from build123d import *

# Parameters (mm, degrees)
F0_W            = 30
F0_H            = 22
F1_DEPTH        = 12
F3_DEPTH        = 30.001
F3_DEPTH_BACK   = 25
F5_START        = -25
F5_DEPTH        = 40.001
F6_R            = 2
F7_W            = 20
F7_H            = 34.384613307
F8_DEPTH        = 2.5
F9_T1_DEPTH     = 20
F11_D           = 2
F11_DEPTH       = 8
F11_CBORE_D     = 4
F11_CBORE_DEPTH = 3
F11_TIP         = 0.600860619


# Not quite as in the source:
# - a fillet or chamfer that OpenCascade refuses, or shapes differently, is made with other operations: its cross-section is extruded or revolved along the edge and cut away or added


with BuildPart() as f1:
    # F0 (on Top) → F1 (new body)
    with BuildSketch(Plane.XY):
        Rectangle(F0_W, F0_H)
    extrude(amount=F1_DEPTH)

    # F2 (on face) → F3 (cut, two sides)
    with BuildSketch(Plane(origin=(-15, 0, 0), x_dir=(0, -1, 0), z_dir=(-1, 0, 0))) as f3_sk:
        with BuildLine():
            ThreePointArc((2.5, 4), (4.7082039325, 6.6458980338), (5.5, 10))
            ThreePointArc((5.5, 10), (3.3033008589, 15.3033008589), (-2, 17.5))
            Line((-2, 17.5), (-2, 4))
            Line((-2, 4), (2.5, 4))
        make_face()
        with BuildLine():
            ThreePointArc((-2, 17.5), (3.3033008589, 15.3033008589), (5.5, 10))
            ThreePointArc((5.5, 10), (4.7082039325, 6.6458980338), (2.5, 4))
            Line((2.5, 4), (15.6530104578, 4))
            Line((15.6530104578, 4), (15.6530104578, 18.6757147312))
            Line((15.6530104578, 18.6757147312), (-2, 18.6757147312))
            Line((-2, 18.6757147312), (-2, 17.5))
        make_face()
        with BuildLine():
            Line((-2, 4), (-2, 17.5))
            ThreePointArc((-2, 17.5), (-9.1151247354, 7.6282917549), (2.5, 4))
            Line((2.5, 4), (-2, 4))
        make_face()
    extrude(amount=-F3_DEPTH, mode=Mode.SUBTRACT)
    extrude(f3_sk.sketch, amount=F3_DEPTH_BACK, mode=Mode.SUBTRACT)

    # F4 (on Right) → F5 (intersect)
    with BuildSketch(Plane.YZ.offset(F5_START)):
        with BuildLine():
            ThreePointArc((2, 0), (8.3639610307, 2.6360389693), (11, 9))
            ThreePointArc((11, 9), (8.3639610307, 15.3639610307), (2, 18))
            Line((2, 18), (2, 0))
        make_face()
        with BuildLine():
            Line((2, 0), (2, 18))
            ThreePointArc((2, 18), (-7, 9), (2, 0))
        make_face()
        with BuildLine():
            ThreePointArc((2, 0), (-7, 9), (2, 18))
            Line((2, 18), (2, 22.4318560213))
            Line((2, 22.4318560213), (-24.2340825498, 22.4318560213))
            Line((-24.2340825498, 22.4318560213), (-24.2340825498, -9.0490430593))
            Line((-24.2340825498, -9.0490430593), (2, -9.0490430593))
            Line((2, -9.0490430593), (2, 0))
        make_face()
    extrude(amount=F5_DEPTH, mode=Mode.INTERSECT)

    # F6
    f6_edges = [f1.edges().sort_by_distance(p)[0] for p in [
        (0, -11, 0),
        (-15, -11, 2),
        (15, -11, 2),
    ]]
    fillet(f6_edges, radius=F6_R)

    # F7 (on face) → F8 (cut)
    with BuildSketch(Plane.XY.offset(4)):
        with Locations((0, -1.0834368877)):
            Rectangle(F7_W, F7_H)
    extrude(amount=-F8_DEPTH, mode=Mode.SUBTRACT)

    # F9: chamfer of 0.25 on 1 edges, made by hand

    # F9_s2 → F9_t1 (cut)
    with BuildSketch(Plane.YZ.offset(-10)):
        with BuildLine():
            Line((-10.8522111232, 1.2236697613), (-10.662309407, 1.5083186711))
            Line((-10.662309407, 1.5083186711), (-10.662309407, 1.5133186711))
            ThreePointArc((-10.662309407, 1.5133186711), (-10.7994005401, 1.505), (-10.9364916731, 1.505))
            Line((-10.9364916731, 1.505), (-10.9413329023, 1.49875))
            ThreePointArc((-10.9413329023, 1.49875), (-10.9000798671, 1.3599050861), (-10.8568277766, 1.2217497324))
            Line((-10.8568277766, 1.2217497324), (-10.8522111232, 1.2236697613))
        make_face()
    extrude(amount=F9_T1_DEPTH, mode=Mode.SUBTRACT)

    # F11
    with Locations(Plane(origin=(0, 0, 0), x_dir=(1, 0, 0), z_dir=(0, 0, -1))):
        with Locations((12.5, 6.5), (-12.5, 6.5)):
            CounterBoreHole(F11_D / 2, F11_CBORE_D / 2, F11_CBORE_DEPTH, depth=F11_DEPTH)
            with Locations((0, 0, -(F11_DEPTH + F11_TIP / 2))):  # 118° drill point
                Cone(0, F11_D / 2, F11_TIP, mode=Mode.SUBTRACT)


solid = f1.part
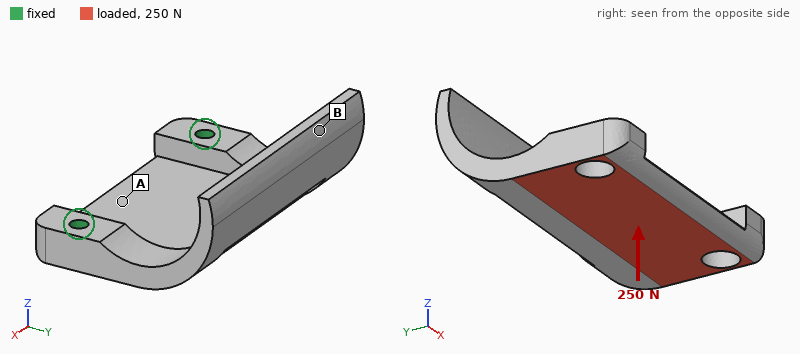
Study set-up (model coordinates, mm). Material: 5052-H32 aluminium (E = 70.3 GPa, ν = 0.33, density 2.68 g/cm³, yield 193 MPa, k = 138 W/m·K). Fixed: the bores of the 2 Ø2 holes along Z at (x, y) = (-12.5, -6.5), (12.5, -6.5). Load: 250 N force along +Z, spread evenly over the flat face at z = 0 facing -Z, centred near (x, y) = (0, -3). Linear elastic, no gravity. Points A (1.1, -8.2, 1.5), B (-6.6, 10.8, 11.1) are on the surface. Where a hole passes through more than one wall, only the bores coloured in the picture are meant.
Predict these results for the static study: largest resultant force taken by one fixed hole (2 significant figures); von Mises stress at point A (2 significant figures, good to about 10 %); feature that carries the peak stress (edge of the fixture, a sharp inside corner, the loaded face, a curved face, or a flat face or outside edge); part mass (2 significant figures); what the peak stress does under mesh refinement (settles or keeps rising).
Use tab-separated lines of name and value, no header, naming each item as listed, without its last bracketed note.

largest resultant force taken by one fixed hole	160 N
von Mises stress at point A	26 MPa
feature that carries the peak stress	edge of the fixture
part mass	3.9 g
what the peak stress does under mesh refinement	keeps rising
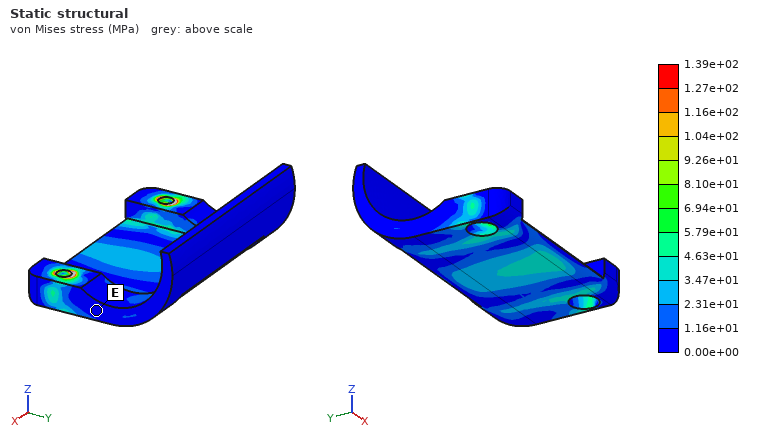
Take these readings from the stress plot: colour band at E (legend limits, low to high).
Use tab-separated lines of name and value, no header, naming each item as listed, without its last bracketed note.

colour band at E	0.00e+00 to 1.16e+01 MPa
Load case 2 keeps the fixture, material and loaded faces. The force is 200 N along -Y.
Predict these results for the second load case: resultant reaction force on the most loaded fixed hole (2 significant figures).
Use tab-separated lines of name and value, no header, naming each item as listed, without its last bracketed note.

resultant reaction force on the most loaded fixed hole	100 N
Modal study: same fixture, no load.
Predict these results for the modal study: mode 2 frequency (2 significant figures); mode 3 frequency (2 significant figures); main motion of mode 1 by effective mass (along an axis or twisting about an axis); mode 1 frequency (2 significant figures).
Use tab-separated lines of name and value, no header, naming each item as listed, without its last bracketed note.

mode 2 frequency	5400 Hz
mode 3 frequency	8300 Hz
main motion of mode 1 by effective mass	along Z
mode 1 frequency	3000 Hz
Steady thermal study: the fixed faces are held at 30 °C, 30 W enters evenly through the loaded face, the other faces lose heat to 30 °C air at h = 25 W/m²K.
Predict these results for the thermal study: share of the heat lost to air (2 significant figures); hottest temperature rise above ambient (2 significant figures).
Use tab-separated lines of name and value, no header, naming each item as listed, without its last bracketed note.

share of the heat lost to air	4.9 %
hottest temperature rise above ambient	51 K
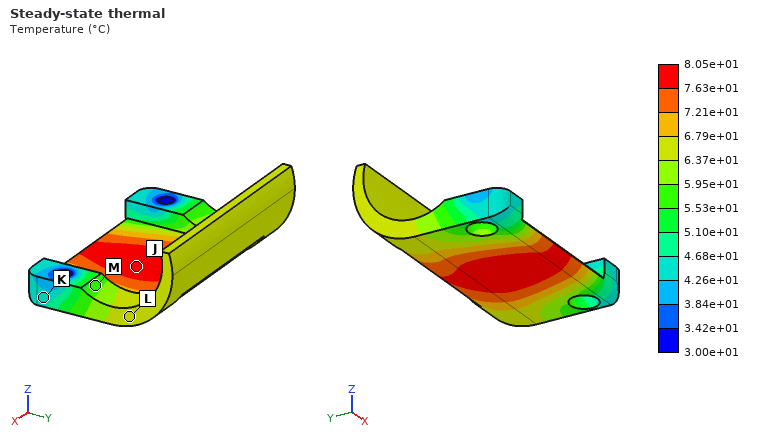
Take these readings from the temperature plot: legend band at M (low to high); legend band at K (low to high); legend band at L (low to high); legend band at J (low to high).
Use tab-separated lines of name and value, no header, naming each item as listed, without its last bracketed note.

legend band at M	5.53e+01 to 5.95e+01 °C
legend band at K	4.26e+01 to 4.68e+01 °C
legend band at L	6.37e+01 to 6.79e+01 °C
legend band at J	7.63e+01 to 8.05e+01 °C
